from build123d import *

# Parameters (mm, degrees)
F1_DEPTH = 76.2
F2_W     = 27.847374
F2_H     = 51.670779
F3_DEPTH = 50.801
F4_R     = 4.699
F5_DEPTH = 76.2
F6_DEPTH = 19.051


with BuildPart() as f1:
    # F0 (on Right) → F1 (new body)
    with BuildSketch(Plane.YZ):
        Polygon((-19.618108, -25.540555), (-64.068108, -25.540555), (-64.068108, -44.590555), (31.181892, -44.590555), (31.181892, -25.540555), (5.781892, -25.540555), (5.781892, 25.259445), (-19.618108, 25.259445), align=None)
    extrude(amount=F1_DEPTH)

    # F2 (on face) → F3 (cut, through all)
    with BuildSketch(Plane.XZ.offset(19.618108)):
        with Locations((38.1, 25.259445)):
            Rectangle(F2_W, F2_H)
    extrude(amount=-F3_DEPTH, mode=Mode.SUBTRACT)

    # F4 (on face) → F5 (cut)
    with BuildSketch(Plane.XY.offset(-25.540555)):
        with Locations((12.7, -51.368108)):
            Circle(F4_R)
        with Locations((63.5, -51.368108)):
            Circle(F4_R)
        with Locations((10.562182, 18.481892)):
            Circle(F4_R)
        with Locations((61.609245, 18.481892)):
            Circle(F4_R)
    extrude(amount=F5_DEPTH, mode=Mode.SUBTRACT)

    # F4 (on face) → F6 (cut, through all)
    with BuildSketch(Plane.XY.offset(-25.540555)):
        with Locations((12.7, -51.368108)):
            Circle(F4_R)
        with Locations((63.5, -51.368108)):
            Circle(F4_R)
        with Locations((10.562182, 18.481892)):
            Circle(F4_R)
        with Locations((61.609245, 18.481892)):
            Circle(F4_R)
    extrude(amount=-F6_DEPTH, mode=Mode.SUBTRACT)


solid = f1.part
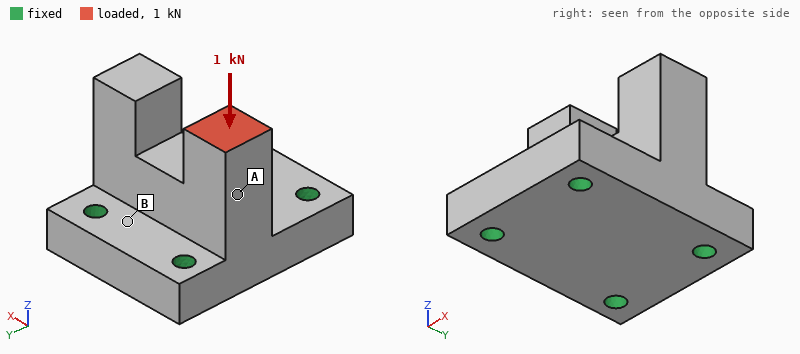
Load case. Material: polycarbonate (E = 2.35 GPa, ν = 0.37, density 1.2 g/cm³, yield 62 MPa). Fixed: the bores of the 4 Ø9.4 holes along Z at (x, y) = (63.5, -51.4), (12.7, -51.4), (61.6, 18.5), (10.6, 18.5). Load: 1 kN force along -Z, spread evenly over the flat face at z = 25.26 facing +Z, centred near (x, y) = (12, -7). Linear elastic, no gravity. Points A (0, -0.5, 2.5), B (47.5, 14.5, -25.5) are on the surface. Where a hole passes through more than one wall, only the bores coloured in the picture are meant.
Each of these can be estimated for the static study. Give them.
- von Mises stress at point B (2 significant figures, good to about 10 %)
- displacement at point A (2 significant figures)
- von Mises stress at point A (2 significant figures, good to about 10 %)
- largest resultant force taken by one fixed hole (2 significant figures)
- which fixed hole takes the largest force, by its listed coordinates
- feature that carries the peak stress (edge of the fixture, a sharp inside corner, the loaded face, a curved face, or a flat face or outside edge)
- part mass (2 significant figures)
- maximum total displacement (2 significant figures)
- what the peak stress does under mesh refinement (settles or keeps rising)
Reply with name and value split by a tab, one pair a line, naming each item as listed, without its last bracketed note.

von Mises stress at point B	0.57 MPa
displacement at point A	0.080 mm
von Mises stress at point A	1.8 MPa
largest resultant force taken by one fixed hole	640 N
which fixed hole takes the largest force, by its listed coordinates	(10.6, 18.5)
feature that carries the peak stress	edge of the fixture
part mass	260 g
maximum total displacement	0.12 mm
what the peak stress does under mesh refinement	keeps rising
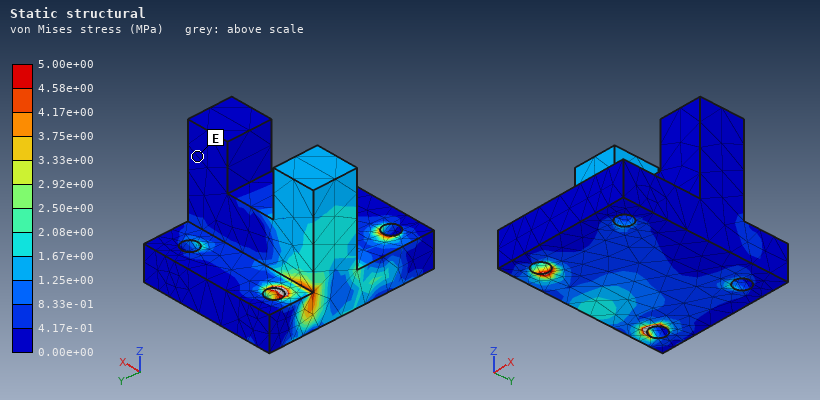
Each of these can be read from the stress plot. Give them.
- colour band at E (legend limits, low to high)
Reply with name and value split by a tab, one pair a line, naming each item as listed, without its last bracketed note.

colour band at E	0.00e+00 to 4.17e-01 MPa
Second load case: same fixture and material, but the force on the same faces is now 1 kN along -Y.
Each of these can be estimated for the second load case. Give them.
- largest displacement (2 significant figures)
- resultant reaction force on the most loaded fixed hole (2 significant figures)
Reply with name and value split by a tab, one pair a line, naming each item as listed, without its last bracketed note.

largest displacement	0.79 mm
resultant reaction force on the most loaded fixed hole	820 N
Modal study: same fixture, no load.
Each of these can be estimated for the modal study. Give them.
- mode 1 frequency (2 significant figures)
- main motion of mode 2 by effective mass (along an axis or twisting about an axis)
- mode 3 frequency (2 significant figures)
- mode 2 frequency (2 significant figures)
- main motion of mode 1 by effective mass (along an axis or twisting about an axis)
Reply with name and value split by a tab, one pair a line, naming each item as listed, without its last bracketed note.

mode 1 frequency	1500 Hz
main motion of mode 2 by effective mass	along X
mode 3 frequency	1900 Hz
mode 2 frequency	1700 Hz
main motion of mode 1 by effective mass	along Y
